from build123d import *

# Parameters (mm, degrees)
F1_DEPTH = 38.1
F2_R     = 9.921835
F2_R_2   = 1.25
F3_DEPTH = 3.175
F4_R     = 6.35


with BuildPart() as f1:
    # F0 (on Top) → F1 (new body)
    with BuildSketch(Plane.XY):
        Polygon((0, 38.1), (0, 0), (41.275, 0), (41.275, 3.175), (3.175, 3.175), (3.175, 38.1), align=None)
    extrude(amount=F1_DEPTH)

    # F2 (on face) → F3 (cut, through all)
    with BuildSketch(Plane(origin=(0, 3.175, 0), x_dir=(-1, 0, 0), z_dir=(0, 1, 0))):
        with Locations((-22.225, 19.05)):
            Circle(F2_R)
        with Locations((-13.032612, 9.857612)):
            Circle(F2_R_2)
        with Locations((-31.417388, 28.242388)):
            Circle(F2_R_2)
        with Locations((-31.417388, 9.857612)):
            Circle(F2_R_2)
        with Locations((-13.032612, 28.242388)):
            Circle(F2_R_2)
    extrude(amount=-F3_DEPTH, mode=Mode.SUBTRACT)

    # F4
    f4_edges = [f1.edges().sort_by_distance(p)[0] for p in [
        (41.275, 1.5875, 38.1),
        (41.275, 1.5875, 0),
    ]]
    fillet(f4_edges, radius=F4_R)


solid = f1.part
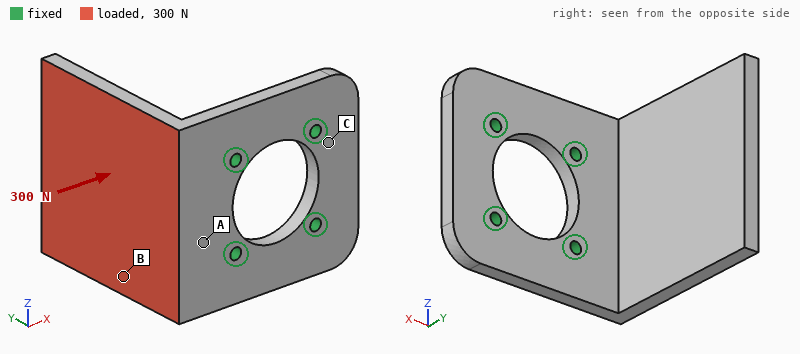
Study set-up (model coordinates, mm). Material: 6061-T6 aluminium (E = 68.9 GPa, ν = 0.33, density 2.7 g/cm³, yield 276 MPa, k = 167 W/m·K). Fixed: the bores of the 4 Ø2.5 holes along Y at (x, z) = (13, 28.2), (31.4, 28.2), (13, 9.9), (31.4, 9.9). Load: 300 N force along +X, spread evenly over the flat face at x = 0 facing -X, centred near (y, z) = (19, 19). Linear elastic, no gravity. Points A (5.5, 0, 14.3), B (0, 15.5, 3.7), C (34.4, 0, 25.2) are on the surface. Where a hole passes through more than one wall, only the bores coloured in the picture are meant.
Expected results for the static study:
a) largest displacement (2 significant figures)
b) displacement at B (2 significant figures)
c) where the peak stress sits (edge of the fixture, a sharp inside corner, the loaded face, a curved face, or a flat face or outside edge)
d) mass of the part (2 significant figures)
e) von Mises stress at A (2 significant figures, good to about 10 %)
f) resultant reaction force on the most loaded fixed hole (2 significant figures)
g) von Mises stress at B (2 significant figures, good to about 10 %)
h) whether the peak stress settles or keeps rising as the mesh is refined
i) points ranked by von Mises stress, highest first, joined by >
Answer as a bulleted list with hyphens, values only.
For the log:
- 0.56 mm
- 0.19 mm
- edge of the fixture
- 22 g
- 70 MPa
- 160 N
- 32 MPa
- keeps rising
- A > B > C
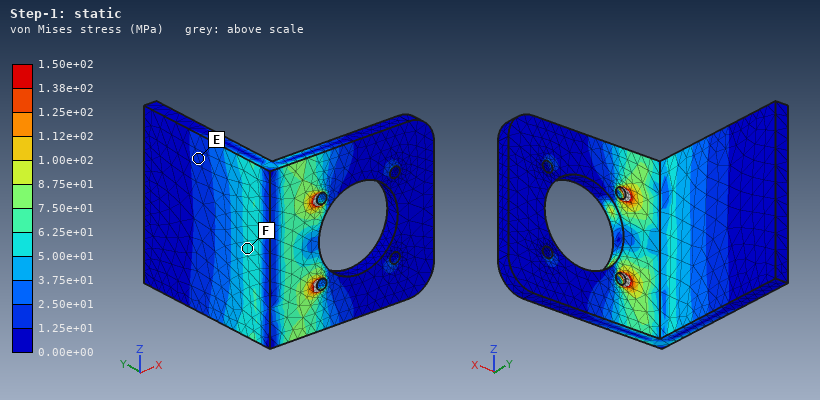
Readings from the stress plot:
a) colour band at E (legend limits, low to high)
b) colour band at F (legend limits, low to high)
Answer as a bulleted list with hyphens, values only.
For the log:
- 1.25e+01 to 2.50e+01 MPa
- 5.00e+01 to 6.25e+01 MPa
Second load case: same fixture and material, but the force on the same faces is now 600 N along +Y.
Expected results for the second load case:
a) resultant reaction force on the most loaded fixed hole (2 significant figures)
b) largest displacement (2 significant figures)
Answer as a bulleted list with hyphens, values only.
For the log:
- 340 N
- 0.38 mm
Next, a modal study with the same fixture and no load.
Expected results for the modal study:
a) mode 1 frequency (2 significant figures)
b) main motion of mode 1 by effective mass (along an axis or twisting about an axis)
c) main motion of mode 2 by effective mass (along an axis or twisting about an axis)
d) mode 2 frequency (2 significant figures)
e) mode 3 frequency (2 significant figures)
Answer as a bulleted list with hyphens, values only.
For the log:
- 1300 Hz
- along X
- along Z
- 2900 Hz
- 4500 Hz
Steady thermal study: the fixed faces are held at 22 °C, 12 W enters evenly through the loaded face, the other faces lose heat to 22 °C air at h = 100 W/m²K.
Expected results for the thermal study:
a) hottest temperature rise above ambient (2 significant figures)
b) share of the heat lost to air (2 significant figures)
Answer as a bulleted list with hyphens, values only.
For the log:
- 14 K
- 21 %
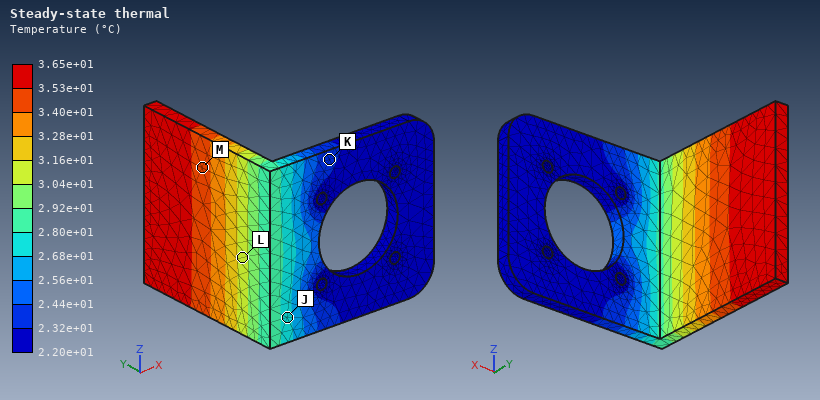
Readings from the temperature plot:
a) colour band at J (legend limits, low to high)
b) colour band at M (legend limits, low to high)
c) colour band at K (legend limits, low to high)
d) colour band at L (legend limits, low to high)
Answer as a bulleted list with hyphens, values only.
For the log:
- 2.68e+01 to 2.80e+01 °C
- 3.40e+01 to 3.53e+01 °C
- 2.32e+01 to 2.44e+01 °C
- 3.04e+01 to 3.16e+01 °C
